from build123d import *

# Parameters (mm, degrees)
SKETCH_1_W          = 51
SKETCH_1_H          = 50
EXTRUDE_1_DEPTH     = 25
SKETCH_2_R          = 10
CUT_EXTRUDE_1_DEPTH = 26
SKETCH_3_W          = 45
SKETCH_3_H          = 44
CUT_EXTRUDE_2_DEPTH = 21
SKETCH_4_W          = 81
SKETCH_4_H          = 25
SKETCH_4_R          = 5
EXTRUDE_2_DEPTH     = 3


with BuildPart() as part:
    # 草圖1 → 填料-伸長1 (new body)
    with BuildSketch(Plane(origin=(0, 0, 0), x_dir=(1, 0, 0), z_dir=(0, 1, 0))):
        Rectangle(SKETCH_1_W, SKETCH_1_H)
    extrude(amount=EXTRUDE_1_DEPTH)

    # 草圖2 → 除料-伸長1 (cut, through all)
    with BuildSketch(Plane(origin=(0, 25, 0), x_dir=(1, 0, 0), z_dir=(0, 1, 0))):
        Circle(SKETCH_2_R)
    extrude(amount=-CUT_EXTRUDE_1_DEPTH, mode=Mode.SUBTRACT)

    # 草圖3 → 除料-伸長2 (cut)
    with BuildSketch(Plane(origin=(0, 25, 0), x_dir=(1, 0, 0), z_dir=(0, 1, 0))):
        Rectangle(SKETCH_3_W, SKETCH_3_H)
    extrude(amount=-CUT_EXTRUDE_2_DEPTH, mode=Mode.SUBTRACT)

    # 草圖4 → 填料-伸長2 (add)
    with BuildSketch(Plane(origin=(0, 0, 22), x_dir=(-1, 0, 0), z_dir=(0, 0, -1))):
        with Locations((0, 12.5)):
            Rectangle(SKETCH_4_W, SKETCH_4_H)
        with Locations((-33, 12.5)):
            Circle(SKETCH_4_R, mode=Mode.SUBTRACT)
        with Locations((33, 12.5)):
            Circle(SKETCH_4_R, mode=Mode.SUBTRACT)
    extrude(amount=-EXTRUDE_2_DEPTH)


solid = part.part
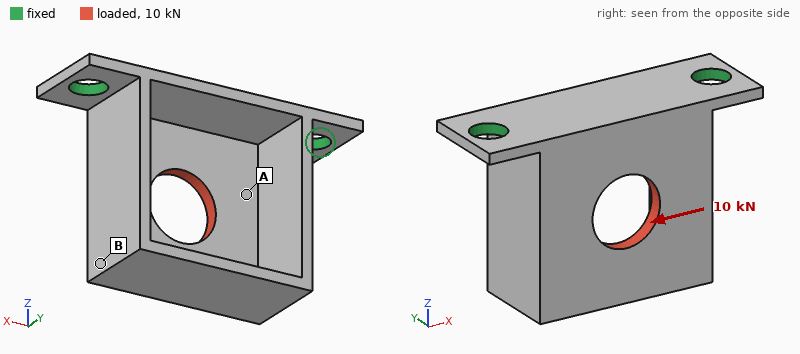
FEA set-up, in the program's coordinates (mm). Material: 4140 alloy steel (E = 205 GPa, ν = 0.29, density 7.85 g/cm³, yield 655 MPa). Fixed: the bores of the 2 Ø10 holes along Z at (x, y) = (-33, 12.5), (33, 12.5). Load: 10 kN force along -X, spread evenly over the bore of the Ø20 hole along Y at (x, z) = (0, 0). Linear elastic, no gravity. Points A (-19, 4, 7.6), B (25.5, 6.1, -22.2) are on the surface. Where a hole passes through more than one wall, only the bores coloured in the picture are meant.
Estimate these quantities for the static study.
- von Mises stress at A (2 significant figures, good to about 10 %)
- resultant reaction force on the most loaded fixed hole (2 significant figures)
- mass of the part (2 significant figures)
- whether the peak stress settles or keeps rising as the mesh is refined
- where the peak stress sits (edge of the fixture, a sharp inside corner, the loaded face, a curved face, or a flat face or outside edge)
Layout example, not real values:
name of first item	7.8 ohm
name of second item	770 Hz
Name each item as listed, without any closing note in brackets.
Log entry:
von Mises stress at A	150 MPa
resultant reaction force on the most loaded fixed hole	6.7 kN
mass of the part	180 g
whether the peak stress settles or keeps rising as the mesh is refined	keeps rising
where the peak stress sits	edge of the fixture
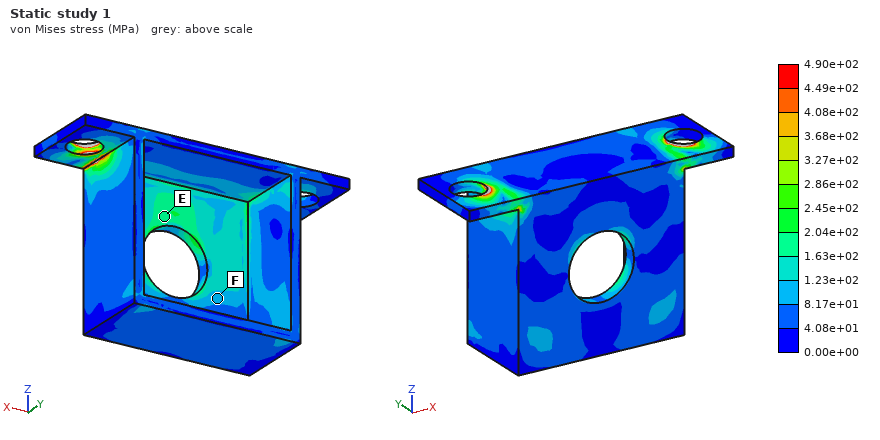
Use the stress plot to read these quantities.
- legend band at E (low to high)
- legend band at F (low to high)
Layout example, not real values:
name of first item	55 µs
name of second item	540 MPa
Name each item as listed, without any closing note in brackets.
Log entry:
legend band at E	1.63e+02 to 2.04e+02 MPa
legend band at F	8.17e+01 to 1.23e+02 MPa
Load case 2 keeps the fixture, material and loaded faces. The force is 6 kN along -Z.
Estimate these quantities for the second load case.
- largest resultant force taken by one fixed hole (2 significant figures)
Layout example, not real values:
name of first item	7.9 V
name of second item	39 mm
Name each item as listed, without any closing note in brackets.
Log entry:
largest resultant force taken by one fixed hole	3.3 kN
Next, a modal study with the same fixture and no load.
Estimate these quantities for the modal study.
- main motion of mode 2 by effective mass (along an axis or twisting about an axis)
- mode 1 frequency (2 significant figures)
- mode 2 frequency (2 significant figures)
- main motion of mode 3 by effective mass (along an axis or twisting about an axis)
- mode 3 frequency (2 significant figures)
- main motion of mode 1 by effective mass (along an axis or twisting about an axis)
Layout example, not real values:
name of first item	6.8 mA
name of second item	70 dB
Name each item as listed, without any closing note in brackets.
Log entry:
main motion of mode 2 by effective mass	along X
mode 1 frequency	1500 Hz
mode 2 frequency	2100 Hz
main motion of mode 3 by effective mass	along Z
mode 3 frequency	6400 Hz
main motion of mode 1 by effective mass	along Y
